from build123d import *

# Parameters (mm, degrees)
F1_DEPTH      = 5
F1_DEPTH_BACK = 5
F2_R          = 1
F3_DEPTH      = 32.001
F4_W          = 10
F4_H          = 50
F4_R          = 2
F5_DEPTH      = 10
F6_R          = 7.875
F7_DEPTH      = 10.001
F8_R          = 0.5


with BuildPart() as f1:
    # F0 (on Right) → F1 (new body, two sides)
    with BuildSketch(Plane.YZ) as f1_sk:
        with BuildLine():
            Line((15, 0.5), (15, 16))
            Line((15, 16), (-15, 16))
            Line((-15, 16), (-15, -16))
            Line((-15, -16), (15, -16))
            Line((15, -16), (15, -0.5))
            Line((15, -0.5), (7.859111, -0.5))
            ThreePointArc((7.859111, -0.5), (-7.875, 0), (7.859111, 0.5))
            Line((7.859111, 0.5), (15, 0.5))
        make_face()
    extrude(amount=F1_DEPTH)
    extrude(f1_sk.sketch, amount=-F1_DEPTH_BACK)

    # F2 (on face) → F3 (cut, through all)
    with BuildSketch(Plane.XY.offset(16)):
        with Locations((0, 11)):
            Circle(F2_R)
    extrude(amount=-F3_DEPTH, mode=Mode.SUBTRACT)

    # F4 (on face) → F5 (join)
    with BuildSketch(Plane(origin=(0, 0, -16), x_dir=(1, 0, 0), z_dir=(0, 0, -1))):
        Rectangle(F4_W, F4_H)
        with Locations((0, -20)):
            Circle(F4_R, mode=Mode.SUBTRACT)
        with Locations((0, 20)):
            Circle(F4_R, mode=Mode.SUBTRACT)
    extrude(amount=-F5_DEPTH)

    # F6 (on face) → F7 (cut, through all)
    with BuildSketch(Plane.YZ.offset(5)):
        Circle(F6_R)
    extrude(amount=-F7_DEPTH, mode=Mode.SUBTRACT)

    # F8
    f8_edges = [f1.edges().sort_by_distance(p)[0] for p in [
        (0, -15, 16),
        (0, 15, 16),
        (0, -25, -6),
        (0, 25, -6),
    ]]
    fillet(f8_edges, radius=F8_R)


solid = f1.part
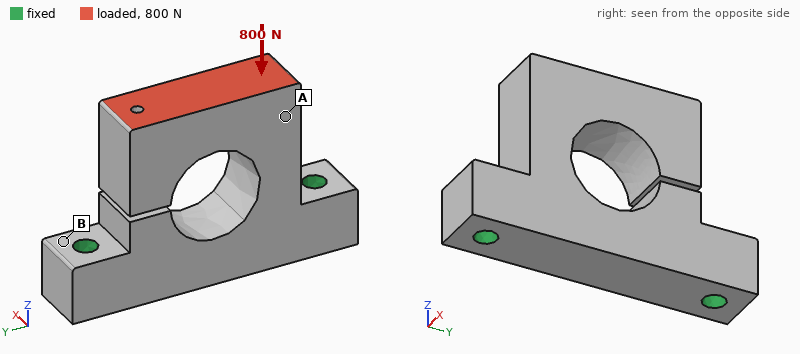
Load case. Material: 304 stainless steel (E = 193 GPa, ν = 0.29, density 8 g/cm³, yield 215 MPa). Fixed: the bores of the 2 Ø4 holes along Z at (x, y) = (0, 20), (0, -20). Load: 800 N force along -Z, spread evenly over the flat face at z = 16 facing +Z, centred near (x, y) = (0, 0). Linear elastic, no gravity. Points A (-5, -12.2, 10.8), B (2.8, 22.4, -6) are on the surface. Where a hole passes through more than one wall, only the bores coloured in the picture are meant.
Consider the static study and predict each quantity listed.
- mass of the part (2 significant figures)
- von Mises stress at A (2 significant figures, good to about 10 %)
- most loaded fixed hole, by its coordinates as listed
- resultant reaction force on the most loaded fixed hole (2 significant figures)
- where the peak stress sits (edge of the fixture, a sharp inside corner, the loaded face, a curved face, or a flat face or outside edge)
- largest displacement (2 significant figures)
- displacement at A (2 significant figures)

74 g
25 MPa
(0, -20)
440 N
a curved face
77 µm
25 µm
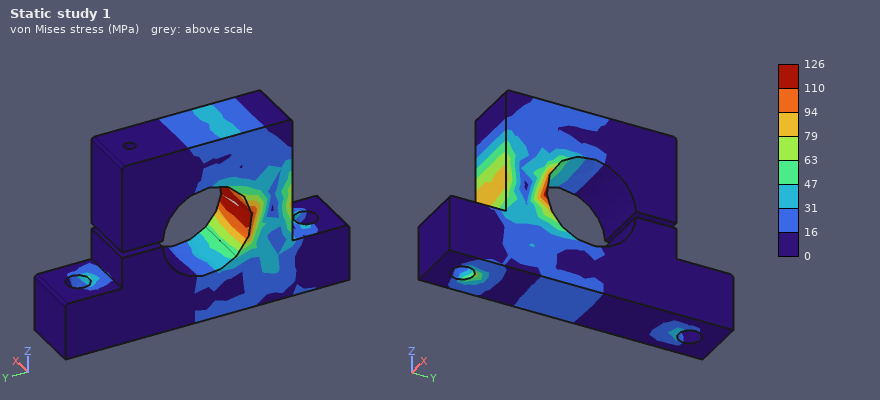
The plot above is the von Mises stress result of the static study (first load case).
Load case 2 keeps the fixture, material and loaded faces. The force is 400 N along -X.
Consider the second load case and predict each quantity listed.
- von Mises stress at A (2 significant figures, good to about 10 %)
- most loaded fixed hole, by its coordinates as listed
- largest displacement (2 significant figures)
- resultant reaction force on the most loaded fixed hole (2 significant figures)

14 MPa
(0, -20)
67 µm
260 N
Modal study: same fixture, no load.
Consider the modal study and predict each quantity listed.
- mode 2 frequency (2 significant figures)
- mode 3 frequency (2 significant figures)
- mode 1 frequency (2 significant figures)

3100 Hz
7400 Hz
3000 Hz
